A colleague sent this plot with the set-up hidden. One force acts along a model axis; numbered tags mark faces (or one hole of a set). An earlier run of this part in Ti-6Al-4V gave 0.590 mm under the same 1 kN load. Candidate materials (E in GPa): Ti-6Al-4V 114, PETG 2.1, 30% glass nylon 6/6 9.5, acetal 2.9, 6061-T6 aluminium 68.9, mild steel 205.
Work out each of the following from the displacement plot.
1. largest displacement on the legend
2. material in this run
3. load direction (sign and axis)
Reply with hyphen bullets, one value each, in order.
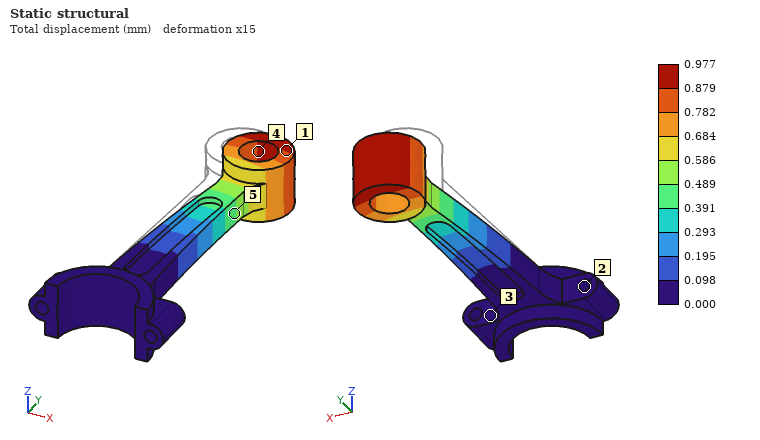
- 0.977 mm
- 6061-T6 aluminium
- +X
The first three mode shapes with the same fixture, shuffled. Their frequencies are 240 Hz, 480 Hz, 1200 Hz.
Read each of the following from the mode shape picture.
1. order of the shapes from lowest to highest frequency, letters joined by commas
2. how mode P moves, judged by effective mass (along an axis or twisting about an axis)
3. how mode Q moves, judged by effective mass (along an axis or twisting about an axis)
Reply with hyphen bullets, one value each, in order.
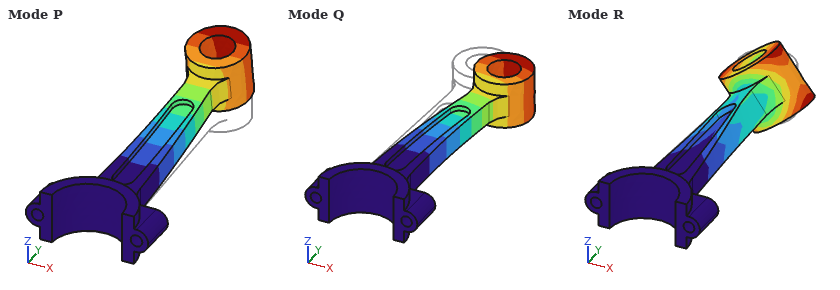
- P, Q, R
- along Z
- along X
